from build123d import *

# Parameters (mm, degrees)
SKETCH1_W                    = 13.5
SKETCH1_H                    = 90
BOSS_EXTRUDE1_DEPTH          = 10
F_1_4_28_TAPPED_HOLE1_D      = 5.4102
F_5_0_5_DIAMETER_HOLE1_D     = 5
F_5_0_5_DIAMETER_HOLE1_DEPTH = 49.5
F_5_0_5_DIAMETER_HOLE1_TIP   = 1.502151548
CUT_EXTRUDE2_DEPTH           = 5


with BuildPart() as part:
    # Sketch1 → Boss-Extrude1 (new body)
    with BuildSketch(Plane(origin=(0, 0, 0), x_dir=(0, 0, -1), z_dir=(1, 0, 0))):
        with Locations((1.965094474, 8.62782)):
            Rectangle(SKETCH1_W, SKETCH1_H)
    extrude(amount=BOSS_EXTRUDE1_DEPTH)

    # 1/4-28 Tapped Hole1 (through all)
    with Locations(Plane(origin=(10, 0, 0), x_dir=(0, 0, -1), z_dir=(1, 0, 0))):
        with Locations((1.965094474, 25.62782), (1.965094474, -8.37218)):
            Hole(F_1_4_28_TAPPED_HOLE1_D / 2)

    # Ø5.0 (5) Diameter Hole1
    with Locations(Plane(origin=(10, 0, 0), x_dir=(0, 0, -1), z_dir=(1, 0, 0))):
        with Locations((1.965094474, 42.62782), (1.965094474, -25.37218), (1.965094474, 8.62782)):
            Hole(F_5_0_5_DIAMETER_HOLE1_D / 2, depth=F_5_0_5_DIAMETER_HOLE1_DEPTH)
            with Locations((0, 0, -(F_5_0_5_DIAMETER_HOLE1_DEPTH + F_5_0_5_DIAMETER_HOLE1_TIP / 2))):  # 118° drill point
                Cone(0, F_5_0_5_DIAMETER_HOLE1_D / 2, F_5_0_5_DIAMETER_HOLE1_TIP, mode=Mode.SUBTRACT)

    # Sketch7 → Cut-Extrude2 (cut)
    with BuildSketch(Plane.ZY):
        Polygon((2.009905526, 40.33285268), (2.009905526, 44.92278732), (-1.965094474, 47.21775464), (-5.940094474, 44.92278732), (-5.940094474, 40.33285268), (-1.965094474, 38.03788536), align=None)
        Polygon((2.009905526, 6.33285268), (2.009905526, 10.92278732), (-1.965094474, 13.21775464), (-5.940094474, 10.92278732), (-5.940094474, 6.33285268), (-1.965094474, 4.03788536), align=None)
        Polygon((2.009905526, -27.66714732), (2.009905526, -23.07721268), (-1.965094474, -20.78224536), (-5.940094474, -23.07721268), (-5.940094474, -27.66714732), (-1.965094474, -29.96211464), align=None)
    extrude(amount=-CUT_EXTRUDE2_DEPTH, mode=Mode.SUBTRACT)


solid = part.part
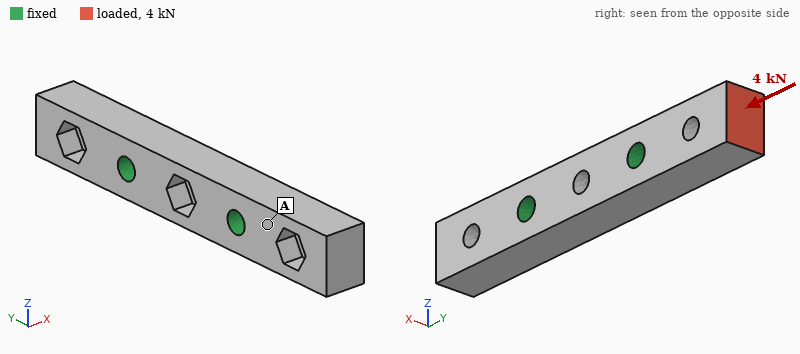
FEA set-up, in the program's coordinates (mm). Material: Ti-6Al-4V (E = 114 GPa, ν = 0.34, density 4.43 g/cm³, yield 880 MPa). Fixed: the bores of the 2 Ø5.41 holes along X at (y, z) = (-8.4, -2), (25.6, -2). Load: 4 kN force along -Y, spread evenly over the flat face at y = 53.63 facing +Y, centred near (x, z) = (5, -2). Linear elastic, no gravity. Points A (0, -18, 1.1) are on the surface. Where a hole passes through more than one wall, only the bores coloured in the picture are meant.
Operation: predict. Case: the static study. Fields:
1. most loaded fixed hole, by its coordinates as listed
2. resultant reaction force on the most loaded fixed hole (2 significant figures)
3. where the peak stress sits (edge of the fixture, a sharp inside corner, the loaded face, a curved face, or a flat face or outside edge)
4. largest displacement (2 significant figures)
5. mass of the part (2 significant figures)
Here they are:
(25.6, -2)
3.9 kN
a curved face
15 µm
47 g
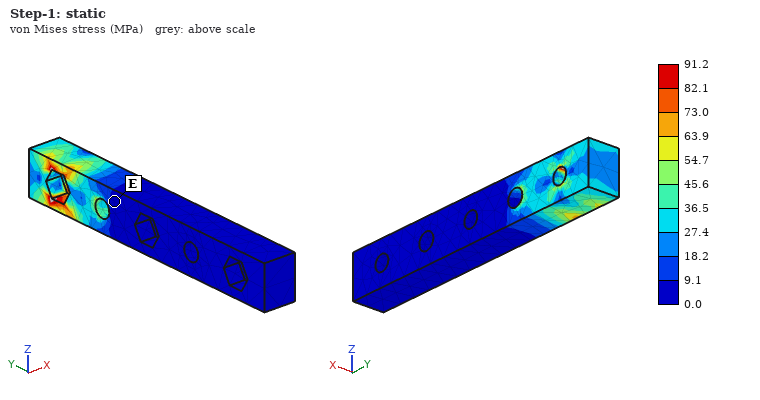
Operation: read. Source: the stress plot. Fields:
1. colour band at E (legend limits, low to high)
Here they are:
0.0 to 9.1 MPa
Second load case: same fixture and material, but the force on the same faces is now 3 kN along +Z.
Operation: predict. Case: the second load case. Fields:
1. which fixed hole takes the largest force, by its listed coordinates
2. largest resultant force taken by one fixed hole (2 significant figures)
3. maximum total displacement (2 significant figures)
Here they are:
(25.6, -2)
3.6 kN
0.16 mm
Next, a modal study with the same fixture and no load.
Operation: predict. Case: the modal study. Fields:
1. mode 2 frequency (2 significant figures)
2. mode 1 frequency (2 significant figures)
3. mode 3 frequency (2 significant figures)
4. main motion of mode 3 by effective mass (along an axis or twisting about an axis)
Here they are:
10 kHz
10 kHz
11 kHz
along Z
